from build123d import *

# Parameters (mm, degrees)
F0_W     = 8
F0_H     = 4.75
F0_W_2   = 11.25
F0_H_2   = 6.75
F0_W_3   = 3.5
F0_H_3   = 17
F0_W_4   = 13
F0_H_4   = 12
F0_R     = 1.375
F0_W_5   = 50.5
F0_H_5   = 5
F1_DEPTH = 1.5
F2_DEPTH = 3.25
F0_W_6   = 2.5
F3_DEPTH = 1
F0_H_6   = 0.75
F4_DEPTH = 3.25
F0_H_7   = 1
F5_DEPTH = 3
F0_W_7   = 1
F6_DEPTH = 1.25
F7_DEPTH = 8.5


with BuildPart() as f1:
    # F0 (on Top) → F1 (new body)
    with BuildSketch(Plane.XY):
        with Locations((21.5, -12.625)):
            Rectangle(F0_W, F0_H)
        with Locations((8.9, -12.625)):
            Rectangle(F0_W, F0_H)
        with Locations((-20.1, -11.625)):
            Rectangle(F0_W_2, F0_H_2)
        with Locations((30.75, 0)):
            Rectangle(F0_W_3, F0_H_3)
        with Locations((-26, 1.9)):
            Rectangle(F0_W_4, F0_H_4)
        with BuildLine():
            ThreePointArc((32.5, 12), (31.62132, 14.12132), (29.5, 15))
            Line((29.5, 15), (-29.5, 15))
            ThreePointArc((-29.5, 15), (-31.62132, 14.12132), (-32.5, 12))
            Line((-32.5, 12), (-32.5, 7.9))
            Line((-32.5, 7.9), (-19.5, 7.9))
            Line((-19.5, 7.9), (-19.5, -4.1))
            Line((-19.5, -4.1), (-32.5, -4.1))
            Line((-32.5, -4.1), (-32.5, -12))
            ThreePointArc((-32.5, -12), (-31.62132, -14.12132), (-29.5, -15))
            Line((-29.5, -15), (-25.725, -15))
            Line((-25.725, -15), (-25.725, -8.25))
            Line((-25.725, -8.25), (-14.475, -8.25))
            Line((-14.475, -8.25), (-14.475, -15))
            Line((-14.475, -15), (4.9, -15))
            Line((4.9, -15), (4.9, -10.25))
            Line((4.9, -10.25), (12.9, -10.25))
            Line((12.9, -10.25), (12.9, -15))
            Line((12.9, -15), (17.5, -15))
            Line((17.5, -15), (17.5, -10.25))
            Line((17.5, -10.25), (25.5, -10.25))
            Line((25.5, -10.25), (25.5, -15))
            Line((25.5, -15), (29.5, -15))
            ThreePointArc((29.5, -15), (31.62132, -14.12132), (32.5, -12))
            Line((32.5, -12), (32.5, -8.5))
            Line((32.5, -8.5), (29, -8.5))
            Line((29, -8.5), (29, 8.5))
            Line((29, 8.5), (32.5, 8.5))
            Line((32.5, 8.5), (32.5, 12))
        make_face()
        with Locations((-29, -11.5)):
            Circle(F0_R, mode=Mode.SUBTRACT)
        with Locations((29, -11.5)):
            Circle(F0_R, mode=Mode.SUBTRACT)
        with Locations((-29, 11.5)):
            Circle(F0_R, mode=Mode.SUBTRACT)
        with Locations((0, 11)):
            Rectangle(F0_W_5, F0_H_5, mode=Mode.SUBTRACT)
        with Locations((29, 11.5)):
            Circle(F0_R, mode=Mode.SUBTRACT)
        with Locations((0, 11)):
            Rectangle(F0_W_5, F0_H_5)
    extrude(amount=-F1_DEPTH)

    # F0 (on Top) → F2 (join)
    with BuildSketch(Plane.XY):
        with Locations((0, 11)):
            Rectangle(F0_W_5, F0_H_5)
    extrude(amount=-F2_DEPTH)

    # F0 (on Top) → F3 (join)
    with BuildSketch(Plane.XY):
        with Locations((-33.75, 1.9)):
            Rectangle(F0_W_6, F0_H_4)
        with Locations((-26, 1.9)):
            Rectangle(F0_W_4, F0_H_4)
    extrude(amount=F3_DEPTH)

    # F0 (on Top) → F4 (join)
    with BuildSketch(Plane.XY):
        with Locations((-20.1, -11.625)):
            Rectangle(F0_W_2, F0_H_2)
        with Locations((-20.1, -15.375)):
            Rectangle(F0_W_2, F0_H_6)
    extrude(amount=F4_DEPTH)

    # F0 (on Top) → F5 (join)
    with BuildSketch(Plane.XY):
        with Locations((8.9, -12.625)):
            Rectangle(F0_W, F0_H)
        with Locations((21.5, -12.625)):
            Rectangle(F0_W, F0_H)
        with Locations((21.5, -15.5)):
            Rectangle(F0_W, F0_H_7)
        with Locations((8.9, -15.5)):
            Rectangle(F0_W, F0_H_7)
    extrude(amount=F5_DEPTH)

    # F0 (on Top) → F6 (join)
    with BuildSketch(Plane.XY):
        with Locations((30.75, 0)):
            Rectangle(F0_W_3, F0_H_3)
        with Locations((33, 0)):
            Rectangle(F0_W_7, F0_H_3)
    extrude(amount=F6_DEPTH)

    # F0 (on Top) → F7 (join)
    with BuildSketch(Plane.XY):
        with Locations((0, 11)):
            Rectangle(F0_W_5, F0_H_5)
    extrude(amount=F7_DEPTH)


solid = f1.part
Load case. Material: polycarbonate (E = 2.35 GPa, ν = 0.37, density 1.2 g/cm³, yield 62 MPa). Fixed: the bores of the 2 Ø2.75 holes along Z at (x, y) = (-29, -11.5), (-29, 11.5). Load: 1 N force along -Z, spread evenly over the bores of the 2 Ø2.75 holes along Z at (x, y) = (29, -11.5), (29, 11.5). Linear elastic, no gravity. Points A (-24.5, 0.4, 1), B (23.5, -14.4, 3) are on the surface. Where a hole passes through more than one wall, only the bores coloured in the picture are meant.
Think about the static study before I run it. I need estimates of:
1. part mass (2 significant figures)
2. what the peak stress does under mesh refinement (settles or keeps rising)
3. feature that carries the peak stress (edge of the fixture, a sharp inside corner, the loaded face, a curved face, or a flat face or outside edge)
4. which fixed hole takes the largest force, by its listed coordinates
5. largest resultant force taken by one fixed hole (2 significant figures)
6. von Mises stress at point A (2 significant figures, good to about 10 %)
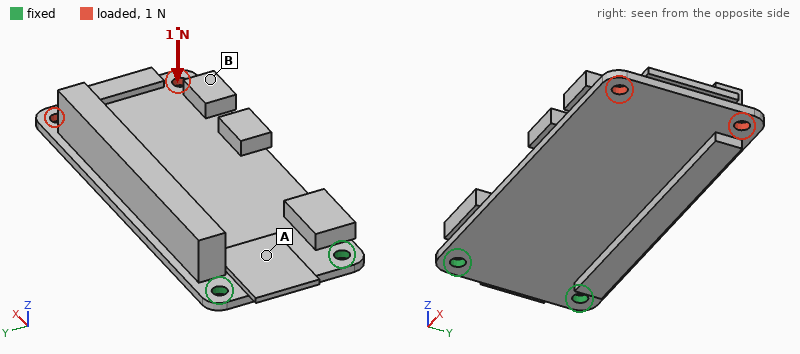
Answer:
7.6 g
keeps rising
edge of the fixture
(-29, -11.5)
1.1 N
1.2 MPa
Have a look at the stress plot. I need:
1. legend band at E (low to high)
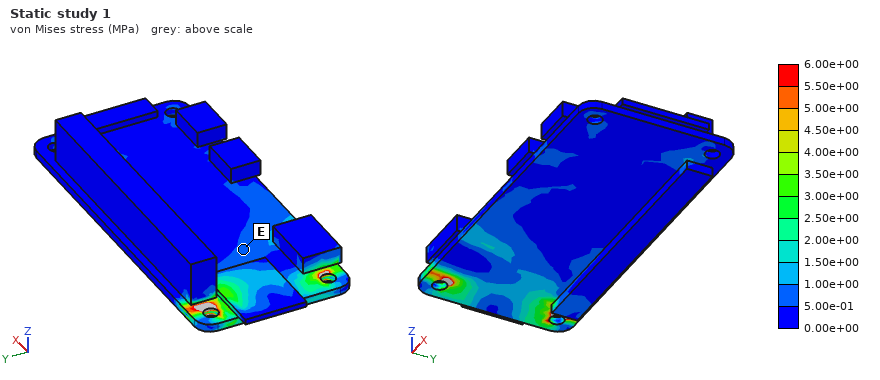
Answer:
5.00e-01 to 1.00e+00 MPa
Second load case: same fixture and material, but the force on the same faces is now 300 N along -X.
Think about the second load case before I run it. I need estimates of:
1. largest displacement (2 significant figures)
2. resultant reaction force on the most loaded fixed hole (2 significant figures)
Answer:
0.56 mm
150 N
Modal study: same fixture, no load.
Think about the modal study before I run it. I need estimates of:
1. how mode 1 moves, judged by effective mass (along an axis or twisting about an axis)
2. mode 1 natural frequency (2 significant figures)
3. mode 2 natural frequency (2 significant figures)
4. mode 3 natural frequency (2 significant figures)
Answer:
along Z
120 Hz
490 Hz
1100 Hz
